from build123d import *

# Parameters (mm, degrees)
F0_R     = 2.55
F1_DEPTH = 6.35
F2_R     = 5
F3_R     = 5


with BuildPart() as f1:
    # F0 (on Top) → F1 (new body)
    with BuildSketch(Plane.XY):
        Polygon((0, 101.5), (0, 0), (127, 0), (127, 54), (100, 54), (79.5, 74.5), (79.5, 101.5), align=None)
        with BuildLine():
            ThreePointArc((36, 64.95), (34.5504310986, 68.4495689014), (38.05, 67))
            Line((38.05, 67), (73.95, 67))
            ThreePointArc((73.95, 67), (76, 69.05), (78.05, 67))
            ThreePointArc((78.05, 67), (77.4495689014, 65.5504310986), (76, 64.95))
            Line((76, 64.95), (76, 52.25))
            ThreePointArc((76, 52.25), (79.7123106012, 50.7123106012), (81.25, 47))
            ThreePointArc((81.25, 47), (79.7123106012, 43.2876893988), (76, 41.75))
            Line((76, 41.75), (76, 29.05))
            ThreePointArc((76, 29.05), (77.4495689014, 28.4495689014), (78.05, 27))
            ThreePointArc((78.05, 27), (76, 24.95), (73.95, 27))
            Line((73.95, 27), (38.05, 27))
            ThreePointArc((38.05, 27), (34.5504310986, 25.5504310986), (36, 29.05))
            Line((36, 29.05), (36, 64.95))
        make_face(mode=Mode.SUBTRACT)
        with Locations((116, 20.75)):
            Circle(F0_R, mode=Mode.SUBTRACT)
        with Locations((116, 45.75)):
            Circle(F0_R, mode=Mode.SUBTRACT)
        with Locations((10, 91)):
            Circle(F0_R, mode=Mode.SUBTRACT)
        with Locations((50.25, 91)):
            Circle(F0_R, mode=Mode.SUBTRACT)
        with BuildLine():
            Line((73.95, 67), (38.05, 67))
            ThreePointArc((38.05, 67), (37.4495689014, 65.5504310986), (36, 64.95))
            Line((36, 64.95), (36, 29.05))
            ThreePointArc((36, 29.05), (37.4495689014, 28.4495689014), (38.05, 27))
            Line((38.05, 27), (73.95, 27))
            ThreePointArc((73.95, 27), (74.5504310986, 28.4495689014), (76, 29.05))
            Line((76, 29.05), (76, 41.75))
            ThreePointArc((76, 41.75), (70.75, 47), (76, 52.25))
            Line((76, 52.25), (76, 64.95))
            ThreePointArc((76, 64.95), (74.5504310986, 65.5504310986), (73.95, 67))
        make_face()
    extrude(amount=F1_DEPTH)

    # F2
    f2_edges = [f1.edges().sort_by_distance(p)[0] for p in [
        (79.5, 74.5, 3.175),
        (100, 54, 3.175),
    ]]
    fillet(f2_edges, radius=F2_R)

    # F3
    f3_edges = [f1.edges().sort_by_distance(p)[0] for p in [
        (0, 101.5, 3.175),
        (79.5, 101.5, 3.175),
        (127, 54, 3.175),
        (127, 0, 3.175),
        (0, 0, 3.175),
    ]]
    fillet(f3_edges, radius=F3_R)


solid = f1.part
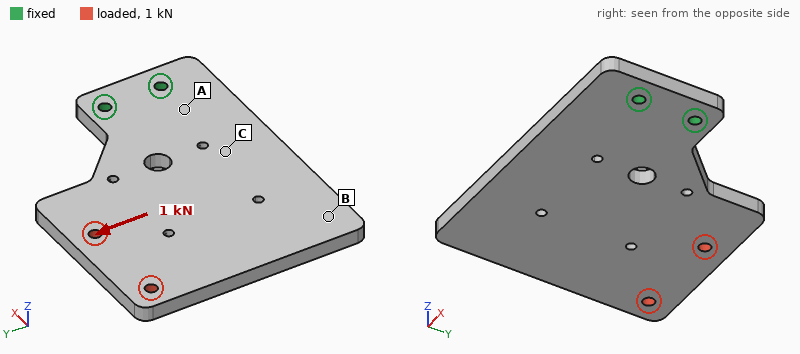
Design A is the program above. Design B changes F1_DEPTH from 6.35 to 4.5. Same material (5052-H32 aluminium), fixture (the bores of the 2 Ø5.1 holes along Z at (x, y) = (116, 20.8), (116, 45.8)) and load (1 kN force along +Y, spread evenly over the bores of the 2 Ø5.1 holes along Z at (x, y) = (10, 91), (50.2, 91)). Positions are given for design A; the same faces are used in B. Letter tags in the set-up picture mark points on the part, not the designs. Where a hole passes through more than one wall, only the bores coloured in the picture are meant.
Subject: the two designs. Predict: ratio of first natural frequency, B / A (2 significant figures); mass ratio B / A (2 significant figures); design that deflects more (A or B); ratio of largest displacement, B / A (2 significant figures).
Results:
0.72
0.71
B
1.4
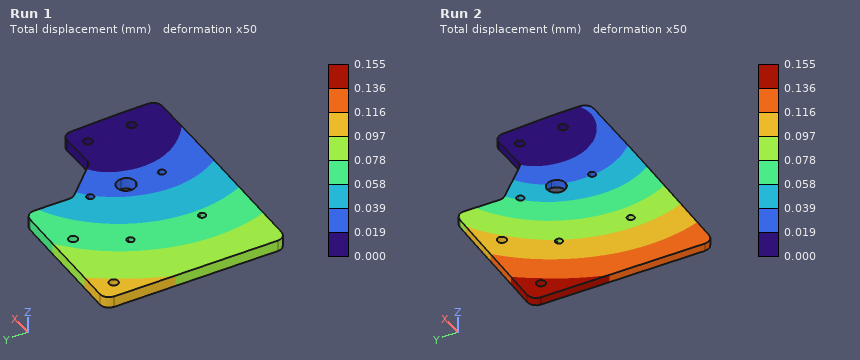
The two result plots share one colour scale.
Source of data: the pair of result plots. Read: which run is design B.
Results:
Run 2
